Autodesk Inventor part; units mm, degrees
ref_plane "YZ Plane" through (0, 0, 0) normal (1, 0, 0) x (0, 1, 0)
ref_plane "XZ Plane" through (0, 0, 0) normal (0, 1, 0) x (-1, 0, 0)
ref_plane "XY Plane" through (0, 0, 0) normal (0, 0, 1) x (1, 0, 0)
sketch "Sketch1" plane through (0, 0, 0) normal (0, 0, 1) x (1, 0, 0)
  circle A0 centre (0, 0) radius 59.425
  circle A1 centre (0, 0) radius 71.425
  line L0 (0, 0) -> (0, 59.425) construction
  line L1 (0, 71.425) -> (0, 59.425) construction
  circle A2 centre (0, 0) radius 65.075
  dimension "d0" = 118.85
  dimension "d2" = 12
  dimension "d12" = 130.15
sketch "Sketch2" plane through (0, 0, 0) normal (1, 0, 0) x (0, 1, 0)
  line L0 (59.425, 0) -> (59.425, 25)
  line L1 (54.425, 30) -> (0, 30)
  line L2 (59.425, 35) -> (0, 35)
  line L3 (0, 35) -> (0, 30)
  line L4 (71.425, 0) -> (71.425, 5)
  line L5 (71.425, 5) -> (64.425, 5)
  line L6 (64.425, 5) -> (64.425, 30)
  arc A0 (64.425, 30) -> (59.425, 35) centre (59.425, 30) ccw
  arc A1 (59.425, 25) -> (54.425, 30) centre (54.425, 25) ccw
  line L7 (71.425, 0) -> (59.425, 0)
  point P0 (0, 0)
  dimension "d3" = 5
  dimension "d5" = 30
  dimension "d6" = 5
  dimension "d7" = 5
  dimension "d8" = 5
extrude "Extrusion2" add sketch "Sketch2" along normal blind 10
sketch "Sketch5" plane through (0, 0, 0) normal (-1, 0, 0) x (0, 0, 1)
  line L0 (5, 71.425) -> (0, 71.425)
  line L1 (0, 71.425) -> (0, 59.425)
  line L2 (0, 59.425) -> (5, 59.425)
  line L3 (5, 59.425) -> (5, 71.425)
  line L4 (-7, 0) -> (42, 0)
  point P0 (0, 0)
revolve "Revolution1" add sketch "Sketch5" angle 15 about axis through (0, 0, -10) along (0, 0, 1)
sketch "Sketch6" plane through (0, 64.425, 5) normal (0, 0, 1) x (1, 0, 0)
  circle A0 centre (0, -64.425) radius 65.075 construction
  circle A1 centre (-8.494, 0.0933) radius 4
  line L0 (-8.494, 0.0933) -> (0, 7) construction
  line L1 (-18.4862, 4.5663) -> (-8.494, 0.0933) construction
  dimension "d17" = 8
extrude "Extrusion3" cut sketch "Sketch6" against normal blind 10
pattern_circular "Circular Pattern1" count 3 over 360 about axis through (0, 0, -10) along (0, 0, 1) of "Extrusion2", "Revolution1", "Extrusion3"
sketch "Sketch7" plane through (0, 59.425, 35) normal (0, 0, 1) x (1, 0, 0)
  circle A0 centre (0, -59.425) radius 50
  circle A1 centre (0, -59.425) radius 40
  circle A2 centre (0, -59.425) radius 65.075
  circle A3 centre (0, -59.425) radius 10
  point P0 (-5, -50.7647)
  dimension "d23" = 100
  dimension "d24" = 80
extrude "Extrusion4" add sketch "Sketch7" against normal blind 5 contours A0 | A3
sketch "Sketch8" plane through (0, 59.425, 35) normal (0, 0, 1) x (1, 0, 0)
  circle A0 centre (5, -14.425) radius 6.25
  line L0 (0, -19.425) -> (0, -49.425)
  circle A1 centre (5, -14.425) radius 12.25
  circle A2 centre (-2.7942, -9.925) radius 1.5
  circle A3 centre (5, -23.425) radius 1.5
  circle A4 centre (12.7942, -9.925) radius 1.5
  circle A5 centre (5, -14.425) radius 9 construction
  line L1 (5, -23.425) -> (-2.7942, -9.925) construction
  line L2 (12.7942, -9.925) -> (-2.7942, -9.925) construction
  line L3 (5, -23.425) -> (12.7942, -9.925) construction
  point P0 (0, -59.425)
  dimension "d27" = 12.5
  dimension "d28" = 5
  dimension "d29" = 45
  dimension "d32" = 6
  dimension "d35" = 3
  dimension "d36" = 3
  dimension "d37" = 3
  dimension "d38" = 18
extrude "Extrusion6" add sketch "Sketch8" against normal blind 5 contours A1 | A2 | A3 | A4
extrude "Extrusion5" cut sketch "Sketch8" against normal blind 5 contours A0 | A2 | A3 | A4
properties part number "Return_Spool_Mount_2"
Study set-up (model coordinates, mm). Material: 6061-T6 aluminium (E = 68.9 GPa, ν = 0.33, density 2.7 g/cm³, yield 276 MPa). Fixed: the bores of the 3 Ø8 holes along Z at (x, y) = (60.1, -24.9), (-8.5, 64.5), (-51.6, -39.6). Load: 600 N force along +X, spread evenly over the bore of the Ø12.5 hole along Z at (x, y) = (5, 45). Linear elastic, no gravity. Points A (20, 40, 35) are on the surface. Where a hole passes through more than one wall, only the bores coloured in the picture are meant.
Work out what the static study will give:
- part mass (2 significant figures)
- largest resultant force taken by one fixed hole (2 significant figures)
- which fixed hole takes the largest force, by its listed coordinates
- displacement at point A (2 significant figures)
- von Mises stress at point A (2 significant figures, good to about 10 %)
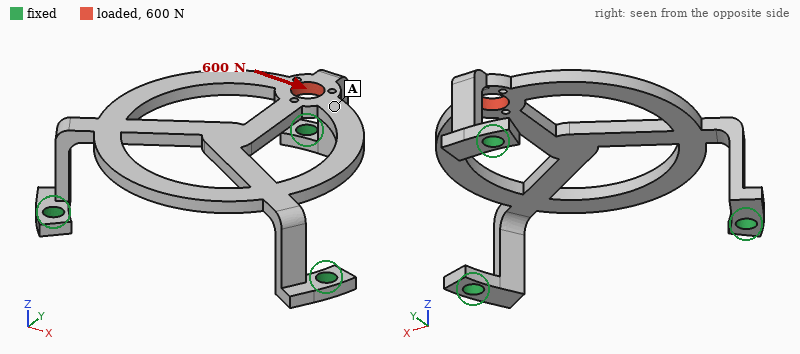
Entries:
82 g
330 N
(-8.5, 64.5)
0.27 mm
19 MPa
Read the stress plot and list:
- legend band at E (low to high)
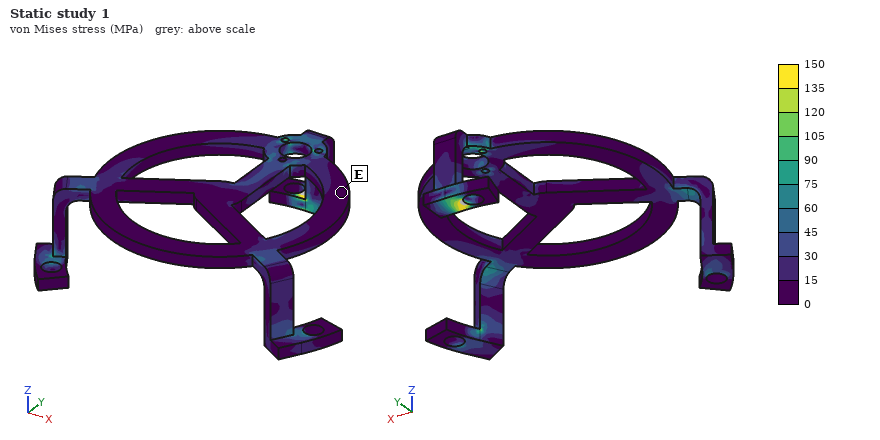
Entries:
0 to 15 MPa
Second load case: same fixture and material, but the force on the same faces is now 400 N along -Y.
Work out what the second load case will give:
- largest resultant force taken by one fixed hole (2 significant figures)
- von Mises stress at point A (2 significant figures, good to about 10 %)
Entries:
160 N
12 MPa
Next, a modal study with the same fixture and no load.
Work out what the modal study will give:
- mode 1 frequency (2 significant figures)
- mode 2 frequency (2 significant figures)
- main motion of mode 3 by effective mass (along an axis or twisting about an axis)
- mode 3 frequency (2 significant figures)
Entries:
1200 Hz
1200 Hz
along Z
1400 Hz
